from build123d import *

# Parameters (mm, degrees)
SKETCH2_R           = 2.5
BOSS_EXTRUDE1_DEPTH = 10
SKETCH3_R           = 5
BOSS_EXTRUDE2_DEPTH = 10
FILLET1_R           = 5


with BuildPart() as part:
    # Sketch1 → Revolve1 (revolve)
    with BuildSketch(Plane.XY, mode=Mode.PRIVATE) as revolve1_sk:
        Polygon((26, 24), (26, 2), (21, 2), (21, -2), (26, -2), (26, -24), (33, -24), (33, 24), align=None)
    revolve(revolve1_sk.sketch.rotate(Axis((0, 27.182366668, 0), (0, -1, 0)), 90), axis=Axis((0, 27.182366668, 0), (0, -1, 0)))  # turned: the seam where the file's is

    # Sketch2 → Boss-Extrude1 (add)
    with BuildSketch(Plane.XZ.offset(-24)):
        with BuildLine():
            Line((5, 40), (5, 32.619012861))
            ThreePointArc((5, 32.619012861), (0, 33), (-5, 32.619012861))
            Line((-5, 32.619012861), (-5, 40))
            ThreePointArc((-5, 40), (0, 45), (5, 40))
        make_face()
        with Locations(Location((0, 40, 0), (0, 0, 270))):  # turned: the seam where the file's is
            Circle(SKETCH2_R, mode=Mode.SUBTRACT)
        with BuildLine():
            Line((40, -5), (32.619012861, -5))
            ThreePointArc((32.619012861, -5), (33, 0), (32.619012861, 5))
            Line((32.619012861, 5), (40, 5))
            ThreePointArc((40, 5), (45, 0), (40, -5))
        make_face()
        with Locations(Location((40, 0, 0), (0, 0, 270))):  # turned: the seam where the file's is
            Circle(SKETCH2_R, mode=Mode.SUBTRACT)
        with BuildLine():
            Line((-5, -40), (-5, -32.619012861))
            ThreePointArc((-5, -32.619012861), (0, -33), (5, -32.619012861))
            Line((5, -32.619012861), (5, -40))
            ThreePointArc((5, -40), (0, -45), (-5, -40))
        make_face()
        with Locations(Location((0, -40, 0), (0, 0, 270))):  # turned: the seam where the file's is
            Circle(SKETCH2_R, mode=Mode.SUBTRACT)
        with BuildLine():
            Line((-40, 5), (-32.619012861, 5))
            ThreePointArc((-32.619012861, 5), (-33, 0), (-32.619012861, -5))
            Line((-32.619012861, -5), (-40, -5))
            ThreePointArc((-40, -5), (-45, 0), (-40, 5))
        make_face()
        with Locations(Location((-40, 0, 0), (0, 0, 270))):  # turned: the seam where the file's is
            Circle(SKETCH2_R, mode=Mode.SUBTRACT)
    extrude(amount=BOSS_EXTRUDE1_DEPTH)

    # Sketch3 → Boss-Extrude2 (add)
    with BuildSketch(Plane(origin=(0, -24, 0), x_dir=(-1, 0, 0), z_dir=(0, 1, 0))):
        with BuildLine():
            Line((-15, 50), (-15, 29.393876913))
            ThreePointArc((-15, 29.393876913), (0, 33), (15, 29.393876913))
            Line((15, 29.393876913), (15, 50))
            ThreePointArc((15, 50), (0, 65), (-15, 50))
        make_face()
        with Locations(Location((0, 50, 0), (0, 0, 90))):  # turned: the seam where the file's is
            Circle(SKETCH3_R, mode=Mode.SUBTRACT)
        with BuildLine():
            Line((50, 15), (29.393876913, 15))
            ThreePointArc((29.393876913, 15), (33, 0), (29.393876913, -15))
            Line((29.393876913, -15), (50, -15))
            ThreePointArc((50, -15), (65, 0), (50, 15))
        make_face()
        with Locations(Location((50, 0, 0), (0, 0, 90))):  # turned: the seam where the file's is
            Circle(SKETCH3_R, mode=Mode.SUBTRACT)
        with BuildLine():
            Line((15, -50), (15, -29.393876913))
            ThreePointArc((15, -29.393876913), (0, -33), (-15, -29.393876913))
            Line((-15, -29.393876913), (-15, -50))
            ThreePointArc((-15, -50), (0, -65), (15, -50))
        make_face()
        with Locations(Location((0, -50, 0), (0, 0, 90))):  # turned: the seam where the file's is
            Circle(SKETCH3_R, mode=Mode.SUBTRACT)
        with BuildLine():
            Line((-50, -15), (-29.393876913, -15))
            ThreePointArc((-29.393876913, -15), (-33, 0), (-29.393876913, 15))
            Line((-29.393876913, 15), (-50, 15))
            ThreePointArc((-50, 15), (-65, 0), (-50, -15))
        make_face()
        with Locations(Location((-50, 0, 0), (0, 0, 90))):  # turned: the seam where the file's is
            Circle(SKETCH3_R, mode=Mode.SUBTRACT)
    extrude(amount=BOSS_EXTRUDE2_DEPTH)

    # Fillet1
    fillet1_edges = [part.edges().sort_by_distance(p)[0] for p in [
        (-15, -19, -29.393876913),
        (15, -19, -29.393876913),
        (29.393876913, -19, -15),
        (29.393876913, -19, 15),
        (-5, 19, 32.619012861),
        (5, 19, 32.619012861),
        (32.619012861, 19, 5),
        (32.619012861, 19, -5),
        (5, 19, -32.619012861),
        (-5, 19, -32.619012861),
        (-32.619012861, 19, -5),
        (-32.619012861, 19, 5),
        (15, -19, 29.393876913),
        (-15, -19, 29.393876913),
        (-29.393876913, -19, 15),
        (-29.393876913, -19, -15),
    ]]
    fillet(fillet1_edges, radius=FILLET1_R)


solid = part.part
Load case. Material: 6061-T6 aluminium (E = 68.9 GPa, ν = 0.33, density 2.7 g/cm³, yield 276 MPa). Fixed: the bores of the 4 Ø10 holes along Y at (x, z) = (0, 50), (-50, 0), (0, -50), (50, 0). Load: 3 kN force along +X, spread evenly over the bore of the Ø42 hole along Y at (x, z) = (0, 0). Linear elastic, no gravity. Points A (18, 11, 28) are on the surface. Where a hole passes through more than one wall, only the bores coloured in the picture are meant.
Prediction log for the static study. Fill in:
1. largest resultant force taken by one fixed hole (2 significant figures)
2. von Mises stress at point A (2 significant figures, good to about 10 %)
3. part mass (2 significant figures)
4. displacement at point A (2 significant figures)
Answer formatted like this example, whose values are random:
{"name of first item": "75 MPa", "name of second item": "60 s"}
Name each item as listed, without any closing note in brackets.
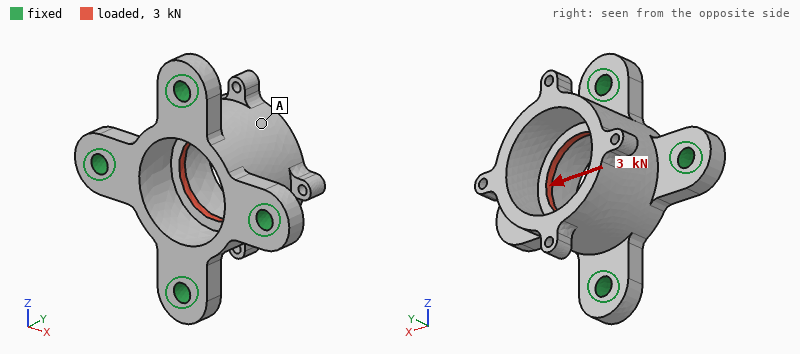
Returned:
{"largest resultant force taken by one fixed hole": "1.2 kN", "von Mises stress at point A": "1.9 MPa", "part mass": "280 g", "displacement at point A": "8.3 µm"}
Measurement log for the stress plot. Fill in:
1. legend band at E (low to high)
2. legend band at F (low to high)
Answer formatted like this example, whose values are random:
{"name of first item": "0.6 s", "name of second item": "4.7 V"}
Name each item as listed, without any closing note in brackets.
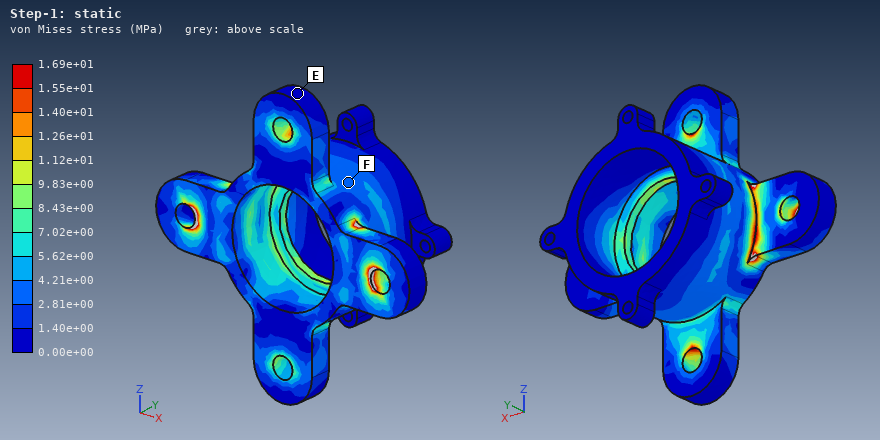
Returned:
{"legend band at E": "0.00e+00 to 1.40e+00 MPa", "legend band at F": "2.81e+00 to 4.21e+00 MPa"}
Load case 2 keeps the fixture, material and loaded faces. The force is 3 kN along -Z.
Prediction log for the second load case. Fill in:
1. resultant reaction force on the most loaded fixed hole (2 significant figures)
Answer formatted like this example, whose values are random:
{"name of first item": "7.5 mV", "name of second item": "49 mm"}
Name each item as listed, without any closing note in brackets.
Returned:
{"resultant reaction force on the most loaded fixed hole": "1.2 kN"}
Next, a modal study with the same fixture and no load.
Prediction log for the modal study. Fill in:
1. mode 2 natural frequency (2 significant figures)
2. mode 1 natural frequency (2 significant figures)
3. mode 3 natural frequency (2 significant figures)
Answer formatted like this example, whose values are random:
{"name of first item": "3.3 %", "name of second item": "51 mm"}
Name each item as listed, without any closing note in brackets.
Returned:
{"mode 2 natural frequency": "6100 Hz", "mode 1 natural frequency": "6100 Hz", "mode 3 natural frequency": "7200 Hz"}
